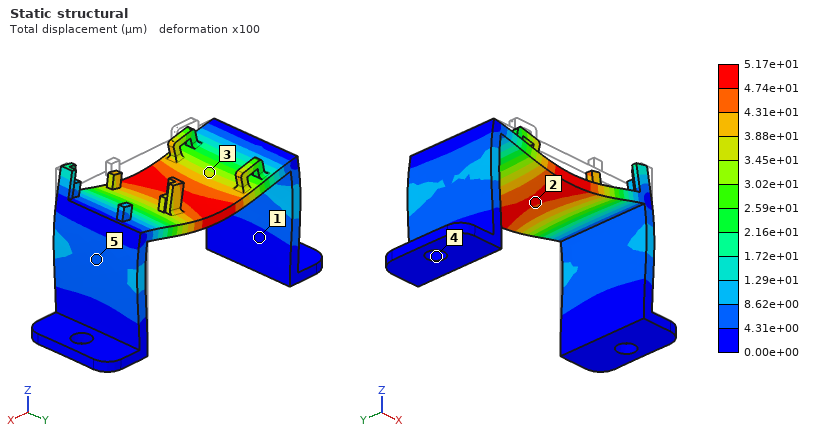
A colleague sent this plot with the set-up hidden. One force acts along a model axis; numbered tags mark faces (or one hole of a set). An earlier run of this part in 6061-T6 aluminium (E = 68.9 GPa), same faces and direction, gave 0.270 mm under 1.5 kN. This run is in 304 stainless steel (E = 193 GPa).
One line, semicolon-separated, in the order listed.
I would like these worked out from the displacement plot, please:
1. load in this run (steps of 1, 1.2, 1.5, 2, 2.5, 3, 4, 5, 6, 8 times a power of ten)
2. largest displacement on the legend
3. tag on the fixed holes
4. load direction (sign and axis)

800 N; 5.17e+01 µm; 4; -Z
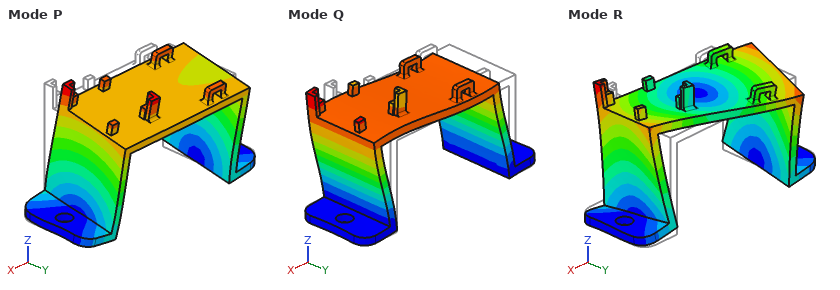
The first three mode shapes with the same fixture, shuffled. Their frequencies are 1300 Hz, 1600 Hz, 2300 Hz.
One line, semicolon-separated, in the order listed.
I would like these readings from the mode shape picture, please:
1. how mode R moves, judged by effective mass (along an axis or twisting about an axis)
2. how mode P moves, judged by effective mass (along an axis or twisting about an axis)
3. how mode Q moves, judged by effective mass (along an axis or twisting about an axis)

twisting about Z; along Y; along X
